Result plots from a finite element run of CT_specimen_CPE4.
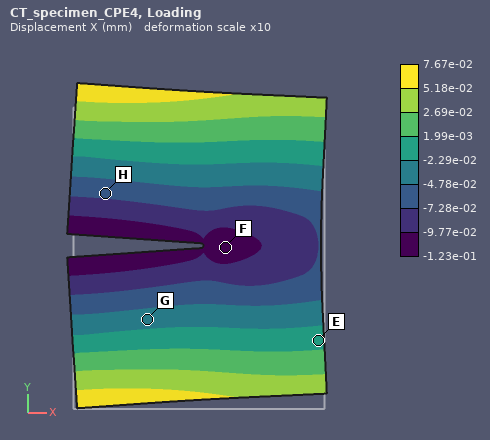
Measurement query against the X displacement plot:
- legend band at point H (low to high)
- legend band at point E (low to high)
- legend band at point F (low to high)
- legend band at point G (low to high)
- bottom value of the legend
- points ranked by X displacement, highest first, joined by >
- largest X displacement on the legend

-7.28e-02 to -4.78e-02 mm
-2.29e-02 to 1.99e-03 mm
-1.23e-01 to -9.77e-02 mm
-4.78e-02 to -2.29e-02 mm
-1.23e-01 mm
E > G > H > F
7.67e-02 mm
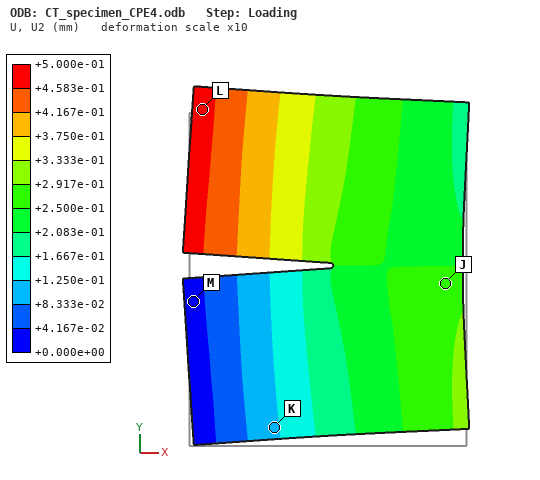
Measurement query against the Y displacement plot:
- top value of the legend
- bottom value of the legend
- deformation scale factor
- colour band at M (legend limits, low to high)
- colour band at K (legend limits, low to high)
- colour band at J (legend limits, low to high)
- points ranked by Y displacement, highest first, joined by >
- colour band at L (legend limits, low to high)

+5.000e-01 mm
+0.000e+00 mm
10
+0.000e+00 to +4.167e-02 mm
+8.333e-02 to +1.250e-01 mm
+2.500e-01 to +2.917e-01 mm
L > J > K > M
+4.583e-01 to +5.000e-01 mm
